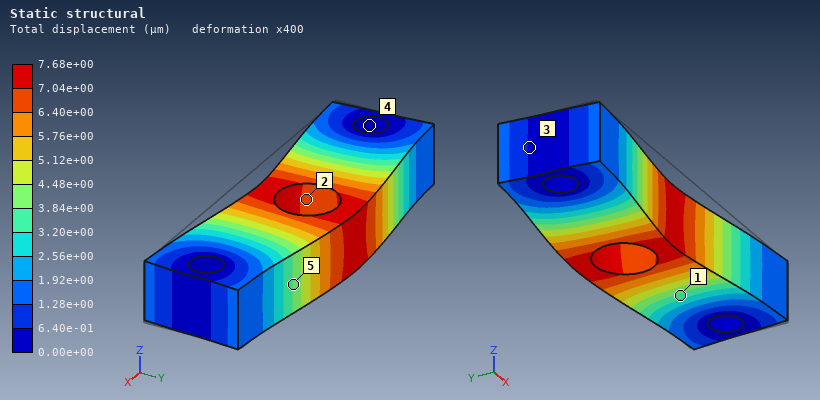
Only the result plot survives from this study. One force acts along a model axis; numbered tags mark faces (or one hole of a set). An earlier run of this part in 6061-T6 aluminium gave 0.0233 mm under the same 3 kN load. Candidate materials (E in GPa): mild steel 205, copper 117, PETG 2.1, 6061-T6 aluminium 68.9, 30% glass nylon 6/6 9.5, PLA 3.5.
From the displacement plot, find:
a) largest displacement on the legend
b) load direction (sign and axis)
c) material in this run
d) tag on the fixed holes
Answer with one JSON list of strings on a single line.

["7.68e+00 µm", "+Y", "mild steel", "4"]
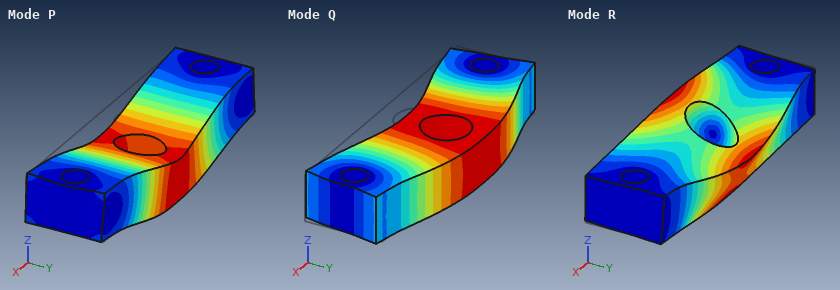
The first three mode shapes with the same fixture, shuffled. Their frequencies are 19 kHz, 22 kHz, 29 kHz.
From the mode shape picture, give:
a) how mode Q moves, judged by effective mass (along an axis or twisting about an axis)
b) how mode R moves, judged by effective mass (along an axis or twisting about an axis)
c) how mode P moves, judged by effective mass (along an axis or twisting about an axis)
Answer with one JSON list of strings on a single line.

["along Y", "twisting about X", "along Z"]
